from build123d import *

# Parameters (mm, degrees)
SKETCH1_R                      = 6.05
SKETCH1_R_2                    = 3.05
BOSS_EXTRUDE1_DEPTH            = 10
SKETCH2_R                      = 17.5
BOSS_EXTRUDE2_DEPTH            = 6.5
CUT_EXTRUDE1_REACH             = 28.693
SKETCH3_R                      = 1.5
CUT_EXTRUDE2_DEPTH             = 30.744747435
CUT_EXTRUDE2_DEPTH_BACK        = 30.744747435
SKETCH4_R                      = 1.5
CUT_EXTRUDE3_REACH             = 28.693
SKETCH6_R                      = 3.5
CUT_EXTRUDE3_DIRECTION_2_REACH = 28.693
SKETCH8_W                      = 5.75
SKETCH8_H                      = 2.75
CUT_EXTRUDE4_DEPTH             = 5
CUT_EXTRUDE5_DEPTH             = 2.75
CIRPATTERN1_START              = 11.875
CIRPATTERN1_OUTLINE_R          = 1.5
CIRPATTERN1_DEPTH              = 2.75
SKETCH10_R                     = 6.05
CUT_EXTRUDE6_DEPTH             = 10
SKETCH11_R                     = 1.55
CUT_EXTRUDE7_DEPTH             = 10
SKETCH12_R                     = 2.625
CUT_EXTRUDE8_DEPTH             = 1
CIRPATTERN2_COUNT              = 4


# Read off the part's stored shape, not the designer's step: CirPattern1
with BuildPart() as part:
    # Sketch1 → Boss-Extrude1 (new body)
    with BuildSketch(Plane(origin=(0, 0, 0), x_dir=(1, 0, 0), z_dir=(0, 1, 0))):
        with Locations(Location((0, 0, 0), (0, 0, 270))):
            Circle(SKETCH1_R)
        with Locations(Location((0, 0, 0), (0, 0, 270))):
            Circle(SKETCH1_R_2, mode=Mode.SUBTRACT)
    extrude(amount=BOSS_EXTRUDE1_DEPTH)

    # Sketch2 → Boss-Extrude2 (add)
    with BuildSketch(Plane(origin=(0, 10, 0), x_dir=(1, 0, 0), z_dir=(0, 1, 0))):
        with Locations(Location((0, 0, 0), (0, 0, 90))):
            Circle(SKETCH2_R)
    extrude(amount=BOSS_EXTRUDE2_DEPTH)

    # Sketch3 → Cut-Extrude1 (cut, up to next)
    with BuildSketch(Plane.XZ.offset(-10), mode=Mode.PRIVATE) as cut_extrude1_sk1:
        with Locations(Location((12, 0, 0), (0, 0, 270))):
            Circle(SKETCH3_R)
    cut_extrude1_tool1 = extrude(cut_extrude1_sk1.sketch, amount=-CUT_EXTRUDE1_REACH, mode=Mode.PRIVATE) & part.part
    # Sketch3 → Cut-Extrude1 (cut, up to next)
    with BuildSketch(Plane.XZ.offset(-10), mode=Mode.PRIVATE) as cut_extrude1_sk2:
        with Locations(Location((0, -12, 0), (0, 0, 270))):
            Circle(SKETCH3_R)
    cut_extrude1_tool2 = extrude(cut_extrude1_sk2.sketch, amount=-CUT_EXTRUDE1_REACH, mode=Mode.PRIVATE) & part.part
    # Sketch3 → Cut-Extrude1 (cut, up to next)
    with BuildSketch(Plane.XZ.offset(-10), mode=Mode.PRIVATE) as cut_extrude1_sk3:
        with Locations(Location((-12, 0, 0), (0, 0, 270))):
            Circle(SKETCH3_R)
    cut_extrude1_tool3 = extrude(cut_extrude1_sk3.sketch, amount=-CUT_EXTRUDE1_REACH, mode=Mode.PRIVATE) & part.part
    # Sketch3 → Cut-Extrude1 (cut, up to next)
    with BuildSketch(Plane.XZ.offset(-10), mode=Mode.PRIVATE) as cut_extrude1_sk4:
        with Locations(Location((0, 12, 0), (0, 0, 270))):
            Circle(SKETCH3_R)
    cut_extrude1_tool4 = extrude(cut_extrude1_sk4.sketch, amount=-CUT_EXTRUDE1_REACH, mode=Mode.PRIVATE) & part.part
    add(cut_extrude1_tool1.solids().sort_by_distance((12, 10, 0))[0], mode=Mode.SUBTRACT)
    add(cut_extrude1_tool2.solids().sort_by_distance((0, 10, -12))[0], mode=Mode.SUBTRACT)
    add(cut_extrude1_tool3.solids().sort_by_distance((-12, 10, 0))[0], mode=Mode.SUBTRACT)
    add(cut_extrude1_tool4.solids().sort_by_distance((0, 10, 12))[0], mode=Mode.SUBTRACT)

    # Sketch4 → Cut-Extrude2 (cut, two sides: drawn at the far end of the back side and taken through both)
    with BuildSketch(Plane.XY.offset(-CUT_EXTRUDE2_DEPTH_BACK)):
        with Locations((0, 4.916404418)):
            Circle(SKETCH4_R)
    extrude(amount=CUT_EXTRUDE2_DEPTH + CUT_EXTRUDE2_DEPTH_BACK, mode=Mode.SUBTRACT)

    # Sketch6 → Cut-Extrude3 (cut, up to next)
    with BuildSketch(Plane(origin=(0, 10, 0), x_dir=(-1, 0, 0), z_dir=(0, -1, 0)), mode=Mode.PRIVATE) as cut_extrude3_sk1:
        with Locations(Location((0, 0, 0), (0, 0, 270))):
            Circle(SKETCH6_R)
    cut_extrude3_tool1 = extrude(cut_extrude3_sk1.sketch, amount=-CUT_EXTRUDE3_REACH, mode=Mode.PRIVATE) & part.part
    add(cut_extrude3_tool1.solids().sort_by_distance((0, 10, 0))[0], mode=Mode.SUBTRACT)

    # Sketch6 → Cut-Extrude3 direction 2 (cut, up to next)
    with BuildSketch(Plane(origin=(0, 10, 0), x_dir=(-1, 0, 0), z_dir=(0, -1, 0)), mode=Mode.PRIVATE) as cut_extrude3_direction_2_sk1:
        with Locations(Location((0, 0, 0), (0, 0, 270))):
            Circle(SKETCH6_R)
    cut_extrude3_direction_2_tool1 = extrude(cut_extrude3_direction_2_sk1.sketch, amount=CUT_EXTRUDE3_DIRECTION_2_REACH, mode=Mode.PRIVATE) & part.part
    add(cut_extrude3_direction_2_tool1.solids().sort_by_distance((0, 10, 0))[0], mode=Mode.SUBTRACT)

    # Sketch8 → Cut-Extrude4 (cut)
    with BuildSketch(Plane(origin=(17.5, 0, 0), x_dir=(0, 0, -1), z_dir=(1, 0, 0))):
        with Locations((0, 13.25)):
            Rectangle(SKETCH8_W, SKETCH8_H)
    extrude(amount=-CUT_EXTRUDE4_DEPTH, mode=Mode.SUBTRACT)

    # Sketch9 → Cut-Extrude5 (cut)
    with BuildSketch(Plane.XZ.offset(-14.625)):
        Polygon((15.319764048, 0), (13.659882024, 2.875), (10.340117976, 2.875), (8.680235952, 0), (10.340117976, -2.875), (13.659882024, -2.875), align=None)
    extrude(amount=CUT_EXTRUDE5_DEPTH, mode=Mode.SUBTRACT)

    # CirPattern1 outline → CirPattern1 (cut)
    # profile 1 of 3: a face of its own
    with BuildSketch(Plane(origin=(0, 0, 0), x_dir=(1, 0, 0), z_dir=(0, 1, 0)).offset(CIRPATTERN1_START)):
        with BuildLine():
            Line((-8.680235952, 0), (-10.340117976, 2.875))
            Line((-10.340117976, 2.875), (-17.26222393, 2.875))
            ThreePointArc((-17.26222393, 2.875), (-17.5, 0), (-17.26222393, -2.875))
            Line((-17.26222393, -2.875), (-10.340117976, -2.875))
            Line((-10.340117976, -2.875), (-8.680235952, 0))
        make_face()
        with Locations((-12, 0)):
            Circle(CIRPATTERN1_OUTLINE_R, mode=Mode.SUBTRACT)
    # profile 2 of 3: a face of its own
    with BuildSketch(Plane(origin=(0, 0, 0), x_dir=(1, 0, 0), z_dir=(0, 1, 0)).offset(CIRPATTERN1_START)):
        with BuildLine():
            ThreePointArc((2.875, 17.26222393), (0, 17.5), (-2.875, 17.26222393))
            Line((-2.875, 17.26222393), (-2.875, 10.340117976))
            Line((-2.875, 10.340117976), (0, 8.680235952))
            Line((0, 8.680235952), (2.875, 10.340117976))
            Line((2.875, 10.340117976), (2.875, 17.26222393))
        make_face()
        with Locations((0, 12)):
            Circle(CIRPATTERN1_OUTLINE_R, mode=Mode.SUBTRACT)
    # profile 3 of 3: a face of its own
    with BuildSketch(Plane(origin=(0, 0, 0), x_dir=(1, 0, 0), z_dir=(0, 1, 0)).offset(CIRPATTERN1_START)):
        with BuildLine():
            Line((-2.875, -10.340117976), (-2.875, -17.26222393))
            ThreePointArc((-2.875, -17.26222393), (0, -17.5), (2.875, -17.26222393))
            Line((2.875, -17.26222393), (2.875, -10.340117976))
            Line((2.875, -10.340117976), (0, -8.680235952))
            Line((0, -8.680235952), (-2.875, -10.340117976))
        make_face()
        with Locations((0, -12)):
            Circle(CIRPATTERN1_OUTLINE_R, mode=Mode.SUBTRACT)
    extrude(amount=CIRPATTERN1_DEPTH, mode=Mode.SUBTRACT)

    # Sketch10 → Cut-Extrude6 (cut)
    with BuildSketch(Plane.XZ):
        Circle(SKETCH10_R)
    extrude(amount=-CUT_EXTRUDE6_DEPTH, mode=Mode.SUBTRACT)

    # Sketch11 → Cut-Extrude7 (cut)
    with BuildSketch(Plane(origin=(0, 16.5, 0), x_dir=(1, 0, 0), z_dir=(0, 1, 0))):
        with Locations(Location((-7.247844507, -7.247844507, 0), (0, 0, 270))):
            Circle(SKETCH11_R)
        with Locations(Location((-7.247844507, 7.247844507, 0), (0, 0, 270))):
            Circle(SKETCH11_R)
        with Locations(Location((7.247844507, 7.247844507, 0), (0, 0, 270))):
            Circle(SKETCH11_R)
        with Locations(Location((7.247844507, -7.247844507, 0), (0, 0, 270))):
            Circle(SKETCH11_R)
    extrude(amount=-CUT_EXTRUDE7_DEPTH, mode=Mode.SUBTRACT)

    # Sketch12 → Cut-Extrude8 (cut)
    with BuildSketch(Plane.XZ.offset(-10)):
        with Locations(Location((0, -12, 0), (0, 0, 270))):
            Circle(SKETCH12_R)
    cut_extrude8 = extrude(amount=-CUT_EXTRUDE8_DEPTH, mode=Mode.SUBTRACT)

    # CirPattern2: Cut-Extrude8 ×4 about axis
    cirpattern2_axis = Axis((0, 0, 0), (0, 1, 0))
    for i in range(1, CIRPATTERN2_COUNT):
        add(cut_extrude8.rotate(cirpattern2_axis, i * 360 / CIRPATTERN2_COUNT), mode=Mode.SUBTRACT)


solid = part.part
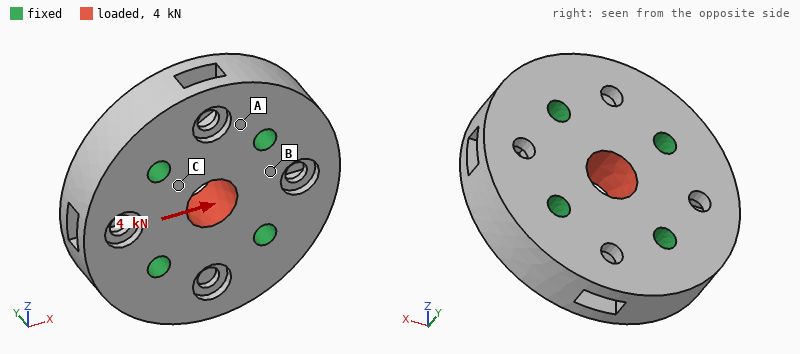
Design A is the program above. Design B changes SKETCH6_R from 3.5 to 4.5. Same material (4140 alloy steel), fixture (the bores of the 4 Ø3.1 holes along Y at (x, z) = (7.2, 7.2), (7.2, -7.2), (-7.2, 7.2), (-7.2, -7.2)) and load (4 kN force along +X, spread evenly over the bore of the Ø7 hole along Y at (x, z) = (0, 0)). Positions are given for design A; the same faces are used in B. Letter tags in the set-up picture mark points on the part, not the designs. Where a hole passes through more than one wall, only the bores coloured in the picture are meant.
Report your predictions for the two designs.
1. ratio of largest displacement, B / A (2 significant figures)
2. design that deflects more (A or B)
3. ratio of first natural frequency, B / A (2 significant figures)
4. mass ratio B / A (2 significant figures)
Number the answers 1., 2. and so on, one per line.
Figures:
1. 0.92
2. A
3. 0.99
4. 0.97
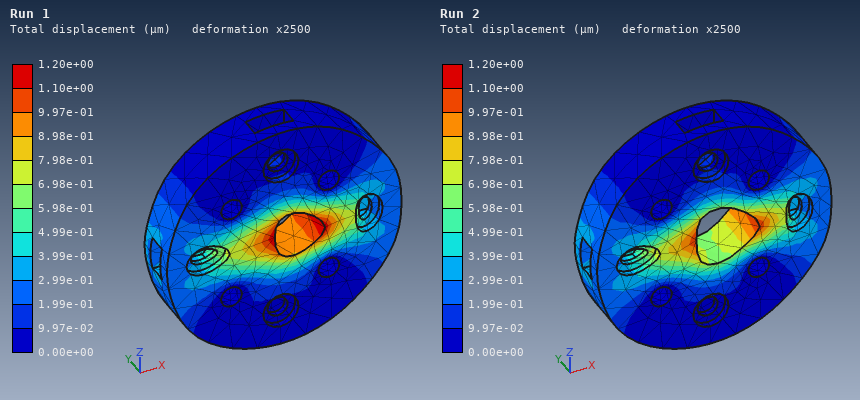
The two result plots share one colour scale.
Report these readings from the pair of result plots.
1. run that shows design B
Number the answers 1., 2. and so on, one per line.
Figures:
1. Run 2
